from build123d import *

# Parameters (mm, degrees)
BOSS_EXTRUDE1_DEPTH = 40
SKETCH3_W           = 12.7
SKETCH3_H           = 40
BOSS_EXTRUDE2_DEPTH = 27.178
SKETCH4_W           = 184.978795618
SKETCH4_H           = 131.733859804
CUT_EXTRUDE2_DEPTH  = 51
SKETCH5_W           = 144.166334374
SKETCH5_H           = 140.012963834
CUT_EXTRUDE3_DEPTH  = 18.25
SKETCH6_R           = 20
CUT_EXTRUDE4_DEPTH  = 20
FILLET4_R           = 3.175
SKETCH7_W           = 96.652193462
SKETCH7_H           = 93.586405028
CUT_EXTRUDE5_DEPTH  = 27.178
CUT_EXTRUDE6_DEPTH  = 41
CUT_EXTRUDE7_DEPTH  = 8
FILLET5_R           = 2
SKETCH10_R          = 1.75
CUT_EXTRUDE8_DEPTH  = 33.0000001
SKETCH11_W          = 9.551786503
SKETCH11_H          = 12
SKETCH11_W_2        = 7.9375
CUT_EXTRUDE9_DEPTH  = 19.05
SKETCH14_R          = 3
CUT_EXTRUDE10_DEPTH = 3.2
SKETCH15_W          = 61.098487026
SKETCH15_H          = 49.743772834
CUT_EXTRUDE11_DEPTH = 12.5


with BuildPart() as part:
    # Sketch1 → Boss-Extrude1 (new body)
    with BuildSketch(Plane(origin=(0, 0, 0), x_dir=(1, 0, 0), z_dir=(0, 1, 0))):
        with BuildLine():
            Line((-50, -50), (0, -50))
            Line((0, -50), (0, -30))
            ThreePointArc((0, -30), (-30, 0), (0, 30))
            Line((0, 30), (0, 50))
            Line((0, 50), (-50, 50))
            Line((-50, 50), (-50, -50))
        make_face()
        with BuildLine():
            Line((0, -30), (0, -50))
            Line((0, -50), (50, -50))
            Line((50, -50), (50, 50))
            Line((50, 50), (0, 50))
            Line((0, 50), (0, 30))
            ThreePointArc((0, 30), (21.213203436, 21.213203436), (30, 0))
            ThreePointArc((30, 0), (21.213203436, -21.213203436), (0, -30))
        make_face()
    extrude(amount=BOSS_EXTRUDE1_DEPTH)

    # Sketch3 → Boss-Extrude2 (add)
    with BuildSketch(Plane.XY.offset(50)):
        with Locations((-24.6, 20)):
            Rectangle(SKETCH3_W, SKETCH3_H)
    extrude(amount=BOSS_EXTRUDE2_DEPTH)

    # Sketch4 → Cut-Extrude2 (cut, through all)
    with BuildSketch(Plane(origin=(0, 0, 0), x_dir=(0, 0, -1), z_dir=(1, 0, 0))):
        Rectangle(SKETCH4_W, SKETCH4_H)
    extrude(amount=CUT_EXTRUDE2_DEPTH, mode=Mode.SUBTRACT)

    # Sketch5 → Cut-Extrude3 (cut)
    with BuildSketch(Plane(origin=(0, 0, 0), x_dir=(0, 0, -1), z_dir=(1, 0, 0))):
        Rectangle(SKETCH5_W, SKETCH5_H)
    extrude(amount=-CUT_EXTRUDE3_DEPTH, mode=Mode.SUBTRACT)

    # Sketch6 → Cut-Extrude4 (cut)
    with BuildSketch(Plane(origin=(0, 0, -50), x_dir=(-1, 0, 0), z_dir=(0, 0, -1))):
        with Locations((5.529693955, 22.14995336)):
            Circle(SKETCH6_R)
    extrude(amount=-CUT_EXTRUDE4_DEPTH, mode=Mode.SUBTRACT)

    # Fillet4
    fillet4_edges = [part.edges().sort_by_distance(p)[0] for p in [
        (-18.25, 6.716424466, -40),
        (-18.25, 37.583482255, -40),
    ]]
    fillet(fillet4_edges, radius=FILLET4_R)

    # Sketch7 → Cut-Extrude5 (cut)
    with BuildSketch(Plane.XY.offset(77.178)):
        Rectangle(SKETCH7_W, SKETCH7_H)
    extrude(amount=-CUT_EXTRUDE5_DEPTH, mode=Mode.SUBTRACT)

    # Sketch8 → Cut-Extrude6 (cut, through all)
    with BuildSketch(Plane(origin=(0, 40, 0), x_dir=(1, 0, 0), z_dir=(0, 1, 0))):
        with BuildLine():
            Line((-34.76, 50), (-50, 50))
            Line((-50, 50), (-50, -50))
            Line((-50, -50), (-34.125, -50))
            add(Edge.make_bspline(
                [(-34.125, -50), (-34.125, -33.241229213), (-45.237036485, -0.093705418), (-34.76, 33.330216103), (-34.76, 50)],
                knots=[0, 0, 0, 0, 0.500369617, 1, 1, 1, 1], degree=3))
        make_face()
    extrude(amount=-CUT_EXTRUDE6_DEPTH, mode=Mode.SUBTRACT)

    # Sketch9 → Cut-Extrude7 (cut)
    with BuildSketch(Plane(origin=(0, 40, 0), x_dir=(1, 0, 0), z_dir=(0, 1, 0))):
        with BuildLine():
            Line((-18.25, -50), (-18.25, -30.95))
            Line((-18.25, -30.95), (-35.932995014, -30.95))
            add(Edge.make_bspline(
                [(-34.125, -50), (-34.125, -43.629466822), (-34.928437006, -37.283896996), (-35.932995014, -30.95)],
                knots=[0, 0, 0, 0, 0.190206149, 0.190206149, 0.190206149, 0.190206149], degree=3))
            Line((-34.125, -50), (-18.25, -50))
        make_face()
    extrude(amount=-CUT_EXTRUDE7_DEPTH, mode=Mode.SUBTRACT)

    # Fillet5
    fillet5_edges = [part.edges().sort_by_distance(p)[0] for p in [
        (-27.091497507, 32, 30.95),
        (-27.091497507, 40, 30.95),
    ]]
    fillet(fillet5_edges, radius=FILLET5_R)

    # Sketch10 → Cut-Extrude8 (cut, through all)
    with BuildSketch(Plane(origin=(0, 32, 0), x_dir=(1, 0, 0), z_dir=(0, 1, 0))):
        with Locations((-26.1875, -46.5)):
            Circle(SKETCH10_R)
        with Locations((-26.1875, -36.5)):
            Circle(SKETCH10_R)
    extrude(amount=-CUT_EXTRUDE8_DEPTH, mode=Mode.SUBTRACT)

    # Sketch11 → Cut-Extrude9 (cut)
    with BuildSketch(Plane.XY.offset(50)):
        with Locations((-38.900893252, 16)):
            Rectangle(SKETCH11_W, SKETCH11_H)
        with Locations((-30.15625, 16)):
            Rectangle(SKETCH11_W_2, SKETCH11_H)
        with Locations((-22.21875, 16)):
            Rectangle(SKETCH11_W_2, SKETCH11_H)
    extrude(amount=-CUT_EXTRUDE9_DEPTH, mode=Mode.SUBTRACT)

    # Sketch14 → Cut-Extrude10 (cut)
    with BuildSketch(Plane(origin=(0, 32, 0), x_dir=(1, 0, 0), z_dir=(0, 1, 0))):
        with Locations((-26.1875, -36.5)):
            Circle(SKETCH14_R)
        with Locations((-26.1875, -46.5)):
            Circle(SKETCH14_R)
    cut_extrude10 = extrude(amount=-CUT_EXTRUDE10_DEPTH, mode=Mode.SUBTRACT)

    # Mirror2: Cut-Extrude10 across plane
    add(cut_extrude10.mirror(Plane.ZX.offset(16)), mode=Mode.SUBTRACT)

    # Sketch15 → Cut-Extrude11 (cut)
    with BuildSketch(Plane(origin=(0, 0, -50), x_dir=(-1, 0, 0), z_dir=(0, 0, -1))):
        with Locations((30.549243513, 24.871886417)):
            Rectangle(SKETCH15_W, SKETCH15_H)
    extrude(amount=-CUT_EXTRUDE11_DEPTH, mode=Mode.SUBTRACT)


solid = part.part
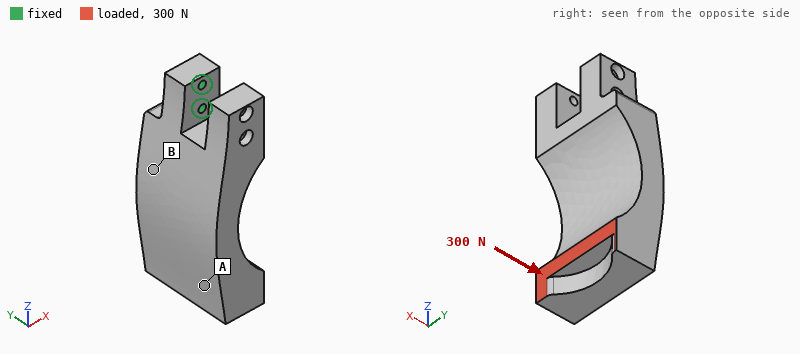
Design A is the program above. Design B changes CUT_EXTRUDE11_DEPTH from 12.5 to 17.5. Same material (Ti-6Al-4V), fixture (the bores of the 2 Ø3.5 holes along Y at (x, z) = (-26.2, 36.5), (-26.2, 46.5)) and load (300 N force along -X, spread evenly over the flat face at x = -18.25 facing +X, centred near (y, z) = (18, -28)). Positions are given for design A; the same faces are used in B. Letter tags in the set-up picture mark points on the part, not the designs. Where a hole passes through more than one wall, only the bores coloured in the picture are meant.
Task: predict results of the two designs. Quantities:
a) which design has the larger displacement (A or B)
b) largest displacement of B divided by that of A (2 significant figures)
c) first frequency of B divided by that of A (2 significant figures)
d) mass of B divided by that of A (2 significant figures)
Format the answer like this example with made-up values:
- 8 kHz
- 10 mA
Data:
- A
- 0.89
- 1.1
- 0.94
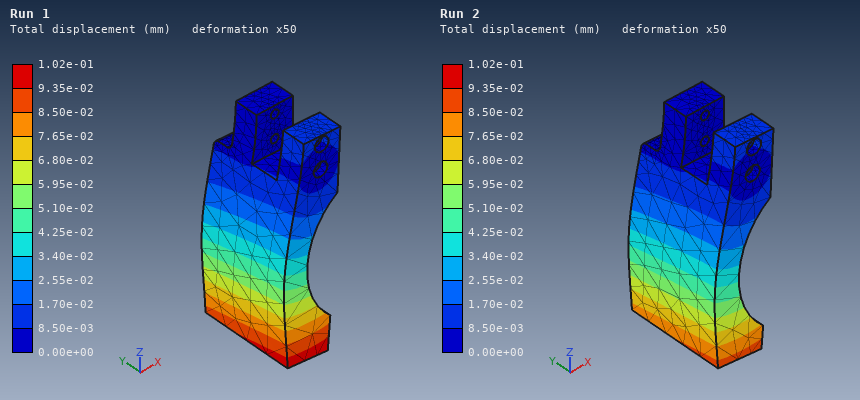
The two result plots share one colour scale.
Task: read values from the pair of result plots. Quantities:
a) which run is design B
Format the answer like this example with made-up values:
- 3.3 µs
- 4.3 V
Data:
- Run 2
